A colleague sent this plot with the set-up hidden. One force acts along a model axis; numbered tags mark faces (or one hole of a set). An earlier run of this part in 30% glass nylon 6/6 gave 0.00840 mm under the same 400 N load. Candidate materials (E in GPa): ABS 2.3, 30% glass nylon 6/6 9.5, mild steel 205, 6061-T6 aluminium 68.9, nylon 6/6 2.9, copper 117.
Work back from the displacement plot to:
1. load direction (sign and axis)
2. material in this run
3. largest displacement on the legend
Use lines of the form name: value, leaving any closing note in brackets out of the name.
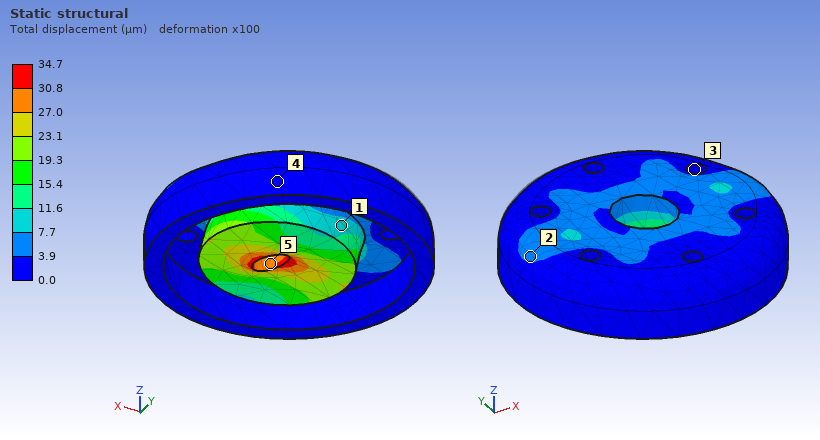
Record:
load direction: +X
material in this run: ABS
largest displacement on the legend: 34.7 µm
